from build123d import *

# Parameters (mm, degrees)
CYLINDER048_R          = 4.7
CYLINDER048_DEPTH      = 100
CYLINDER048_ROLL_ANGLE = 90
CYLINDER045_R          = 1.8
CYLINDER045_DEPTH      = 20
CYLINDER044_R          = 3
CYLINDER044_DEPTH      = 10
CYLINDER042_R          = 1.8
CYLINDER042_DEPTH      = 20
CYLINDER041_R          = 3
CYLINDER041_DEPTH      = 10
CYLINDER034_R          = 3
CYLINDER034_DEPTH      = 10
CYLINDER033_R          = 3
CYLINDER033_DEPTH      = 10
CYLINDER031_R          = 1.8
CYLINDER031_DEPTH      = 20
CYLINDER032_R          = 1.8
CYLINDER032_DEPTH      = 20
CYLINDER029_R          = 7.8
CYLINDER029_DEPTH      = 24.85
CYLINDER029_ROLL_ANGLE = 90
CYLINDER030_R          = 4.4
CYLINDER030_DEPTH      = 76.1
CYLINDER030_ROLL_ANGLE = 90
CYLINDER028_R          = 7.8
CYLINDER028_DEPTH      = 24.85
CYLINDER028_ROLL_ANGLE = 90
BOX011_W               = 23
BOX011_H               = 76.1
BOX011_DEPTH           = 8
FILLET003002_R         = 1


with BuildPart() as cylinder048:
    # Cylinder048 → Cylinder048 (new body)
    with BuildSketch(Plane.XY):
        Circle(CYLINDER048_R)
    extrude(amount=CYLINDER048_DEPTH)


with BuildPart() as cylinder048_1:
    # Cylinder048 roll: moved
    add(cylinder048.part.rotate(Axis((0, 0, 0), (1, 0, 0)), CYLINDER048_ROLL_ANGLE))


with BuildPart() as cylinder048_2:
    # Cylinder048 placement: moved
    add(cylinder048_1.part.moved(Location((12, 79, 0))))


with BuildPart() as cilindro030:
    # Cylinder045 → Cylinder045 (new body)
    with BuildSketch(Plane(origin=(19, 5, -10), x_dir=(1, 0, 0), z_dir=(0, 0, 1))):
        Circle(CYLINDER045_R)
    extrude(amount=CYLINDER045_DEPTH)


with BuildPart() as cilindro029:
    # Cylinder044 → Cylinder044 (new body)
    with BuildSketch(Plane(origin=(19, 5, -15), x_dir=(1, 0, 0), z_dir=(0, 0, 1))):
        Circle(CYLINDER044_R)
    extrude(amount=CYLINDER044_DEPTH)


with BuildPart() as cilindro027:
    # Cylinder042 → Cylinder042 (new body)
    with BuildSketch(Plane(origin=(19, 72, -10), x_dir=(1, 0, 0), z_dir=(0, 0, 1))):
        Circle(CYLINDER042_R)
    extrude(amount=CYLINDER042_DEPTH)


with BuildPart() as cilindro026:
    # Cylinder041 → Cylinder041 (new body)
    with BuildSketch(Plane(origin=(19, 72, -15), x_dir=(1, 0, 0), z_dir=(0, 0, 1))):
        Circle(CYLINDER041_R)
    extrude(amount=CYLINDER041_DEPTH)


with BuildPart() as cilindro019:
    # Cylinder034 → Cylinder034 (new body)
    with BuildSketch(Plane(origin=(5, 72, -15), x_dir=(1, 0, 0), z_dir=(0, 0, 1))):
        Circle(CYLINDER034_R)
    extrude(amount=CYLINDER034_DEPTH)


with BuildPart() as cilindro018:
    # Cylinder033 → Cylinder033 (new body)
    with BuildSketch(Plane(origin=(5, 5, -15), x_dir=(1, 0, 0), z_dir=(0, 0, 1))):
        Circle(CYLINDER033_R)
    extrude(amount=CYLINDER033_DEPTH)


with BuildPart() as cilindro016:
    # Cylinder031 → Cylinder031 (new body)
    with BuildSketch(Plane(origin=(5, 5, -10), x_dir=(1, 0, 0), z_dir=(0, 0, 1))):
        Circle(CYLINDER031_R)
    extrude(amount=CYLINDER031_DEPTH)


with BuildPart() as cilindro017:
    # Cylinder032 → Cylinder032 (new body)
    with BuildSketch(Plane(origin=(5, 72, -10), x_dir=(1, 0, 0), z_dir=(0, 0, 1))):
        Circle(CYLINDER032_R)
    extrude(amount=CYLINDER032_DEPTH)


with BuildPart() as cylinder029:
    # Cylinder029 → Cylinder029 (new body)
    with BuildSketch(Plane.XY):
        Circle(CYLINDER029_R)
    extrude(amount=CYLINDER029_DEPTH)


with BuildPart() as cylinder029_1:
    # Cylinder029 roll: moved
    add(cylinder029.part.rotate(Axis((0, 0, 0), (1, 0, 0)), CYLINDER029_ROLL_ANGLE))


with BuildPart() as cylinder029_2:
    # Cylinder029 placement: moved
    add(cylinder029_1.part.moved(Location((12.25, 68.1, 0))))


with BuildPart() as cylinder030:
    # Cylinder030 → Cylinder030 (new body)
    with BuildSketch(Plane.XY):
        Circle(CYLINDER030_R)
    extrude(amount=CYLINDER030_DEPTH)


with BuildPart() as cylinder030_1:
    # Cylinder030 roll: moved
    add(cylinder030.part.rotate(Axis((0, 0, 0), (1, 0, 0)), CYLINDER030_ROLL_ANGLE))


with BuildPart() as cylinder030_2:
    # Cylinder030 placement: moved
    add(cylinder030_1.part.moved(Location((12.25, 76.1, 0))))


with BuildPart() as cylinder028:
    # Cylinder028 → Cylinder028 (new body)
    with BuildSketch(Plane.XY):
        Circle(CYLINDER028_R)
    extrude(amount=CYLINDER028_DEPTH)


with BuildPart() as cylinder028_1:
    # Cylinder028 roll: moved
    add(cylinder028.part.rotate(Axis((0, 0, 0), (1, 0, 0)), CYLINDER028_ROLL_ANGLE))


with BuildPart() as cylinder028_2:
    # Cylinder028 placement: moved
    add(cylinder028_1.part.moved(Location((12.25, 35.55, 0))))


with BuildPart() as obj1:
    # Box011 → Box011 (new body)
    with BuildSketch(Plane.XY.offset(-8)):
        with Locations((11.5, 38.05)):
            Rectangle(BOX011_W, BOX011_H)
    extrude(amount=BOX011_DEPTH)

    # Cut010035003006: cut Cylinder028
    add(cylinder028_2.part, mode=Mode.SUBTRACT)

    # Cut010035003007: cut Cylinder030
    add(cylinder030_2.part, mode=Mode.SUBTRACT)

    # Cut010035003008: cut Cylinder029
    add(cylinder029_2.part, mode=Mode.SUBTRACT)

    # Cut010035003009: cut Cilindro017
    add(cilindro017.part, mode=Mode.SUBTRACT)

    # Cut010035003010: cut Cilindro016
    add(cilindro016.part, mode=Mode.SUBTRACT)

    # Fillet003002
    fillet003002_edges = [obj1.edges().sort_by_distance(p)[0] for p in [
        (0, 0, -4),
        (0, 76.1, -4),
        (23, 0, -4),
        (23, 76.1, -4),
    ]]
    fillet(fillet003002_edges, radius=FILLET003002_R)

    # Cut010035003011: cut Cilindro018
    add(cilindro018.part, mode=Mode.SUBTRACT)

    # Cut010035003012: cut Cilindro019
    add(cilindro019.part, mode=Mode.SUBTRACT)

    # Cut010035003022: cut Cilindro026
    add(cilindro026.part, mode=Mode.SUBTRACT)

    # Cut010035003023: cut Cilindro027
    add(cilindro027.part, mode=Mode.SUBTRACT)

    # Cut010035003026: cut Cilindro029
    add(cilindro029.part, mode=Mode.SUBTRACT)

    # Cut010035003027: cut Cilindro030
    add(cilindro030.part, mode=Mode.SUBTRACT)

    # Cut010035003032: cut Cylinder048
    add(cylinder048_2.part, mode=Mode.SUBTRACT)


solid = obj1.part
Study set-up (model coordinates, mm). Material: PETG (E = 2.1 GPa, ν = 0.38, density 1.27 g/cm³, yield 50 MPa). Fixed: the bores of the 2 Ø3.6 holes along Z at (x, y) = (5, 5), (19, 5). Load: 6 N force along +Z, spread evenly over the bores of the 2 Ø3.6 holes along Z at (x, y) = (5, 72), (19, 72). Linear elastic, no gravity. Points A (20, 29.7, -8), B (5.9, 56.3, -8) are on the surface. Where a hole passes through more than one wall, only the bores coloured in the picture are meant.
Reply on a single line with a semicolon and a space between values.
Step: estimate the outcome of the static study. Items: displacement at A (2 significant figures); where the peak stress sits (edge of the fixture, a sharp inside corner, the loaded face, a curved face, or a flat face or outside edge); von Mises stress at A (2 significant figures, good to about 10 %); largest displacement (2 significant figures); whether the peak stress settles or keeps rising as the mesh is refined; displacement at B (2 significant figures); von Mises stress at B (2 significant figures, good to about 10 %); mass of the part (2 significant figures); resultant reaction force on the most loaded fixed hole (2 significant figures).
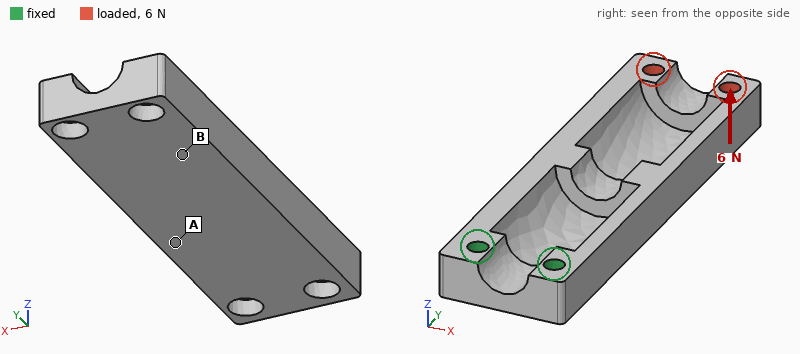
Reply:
0.14 mm; edge of the fixture; 1.6 MPa; 0.72 mm; keeps rising; 0.44 mm; 0.63 MPa; 9.9 g; 5.3 N
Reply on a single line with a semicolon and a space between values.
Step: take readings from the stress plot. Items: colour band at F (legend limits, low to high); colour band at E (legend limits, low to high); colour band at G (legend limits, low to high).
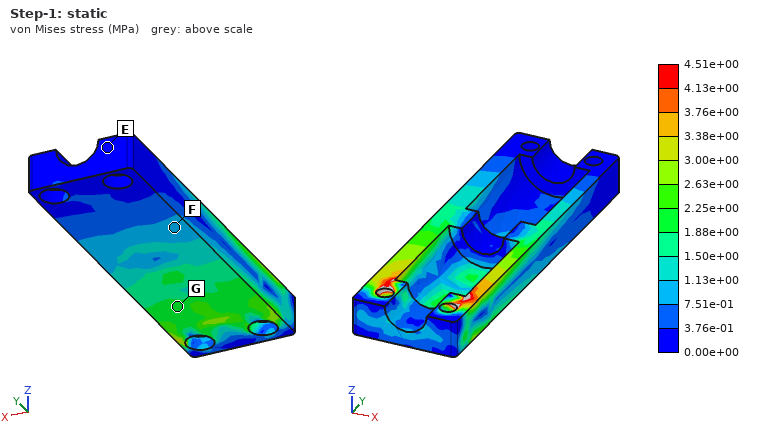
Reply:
7.51e-01 to 1.13e+00 MPa; 0.00e+00 to 3.76e-01 MPa; 1.88e+00 to 2.25e+00 MPa
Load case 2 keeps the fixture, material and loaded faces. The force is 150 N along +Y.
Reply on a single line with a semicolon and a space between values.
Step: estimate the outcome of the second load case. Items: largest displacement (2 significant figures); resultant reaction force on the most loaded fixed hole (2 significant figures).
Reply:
0.82 mm; 75 N
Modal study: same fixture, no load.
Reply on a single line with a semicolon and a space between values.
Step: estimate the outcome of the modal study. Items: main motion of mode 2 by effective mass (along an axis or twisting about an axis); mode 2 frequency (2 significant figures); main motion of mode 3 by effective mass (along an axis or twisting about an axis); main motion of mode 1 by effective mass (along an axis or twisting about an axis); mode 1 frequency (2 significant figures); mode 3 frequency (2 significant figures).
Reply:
along X; 650 Hz; along X; along Z; 290 Hz; 1100 Hz
